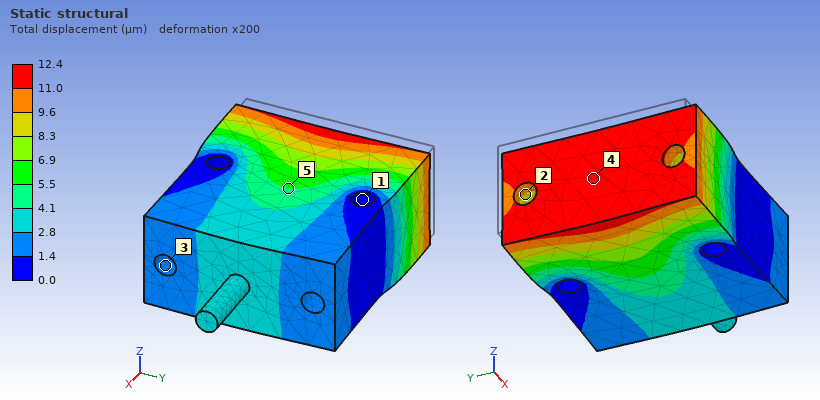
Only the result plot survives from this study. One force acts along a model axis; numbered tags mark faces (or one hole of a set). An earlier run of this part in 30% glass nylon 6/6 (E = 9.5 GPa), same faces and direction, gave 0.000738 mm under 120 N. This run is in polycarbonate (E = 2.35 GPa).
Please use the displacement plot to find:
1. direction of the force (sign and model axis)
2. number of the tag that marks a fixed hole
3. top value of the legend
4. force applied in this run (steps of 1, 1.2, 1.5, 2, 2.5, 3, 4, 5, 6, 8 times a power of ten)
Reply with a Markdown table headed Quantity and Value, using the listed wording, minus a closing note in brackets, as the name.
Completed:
| Quantity | Value |
|---|---|
| direction of the force | +X |
| number of the tag that marks a fixed hole | 1 |
| top value of the legend | 12.4 µm |
| force applied in this run | 500 N |
